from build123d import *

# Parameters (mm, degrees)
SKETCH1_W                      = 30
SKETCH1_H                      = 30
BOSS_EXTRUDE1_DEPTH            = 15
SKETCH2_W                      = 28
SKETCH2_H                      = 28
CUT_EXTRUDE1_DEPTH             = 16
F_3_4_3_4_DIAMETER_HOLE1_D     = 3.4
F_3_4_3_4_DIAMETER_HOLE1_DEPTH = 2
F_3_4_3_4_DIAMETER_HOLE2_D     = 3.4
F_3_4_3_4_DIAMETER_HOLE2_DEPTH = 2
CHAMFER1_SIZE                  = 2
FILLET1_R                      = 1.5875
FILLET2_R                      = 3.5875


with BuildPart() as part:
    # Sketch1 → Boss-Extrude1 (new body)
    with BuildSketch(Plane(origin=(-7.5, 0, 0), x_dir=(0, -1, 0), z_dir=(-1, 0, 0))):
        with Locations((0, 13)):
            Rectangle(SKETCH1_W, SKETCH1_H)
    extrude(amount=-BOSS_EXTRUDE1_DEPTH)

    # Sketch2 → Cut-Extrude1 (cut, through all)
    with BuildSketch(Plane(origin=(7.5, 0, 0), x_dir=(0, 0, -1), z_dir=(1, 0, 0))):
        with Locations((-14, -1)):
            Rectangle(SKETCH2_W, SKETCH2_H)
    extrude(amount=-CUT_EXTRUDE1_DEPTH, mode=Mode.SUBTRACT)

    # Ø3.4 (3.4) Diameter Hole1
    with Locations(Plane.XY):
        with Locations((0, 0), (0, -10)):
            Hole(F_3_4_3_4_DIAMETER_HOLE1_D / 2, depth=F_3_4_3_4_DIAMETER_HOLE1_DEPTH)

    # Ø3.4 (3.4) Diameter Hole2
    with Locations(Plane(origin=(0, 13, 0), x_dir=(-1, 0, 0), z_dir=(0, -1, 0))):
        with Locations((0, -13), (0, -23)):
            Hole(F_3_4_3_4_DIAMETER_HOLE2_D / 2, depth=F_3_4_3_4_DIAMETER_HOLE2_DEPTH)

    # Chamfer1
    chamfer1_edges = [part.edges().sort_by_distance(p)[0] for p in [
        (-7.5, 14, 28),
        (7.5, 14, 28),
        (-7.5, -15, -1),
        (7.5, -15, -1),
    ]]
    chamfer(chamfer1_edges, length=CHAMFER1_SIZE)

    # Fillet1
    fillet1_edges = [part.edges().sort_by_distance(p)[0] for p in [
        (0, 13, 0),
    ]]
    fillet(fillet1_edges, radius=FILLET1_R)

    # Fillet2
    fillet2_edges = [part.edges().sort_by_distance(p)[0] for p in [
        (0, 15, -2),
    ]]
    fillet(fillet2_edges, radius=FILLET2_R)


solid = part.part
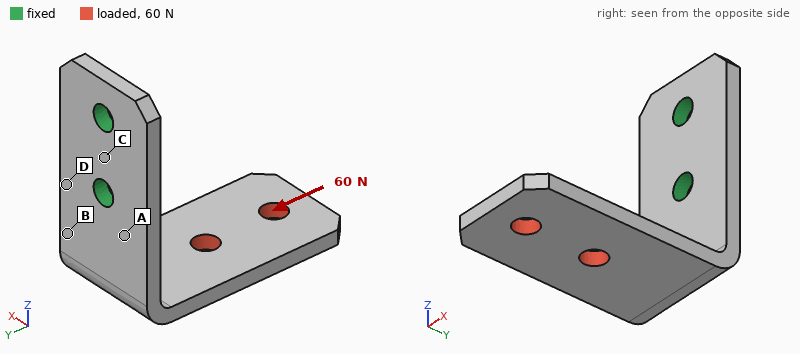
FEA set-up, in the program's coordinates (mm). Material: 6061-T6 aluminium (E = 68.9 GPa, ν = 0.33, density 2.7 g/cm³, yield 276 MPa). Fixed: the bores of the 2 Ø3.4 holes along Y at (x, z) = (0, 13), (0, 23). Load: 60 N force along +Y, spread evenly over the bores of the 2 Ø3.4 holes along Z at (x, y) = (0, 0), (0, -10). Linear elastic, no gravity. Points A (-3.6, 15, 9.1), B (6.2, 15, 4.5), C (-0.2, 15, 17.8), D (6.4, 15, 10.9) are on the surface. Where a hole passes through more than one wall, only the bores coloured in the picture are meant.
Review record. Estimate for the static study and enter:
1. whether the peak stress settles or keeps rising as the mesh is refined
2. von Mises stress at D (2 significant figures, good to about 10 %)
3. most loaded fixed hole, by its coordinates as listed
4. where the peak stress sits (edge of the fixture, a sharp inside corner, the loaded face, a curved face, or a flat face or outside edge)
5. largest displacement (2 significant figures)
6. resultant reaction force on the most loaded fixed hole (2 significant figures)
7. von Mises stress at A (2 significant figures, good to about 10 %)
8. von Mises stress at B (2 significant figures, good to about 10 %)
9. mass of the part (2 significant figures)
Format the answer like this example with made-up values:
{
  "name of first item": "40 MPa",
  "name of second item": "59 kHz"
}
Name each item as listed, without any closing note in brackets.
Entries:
{
  "whether the peak stress settles or keeps rising as the mesh is refined": "keeps rising",
  "von Mises stress at D": "45 MPa",
  "most loaded fixed hole, by its coordinates as listed": "(0, 13)",
  "where the peak stress sits": "edge of the fixture",
  "largest displacement": "0.23 mm",
  "resultant reaction force on the most loaded fixed hole": "77 N",
  "von Mises stress at A": "54 MPa",
  "von Mises stress at B": "33 MPa",
  "mass of the part": "4.4 g"
}
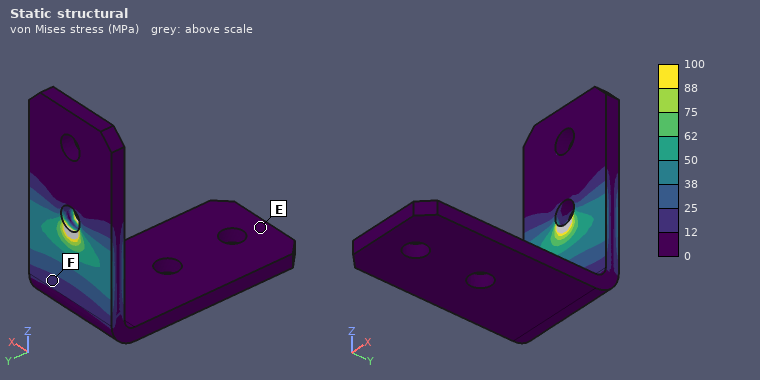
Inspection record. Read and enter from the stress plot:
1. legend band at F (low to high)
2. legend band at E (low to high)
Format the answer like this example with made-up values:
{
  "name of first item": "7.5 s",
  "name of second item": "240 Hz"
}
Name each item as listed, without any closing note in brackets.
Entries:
{
  "legend band at F": "12 to 25 MPa",
  "legend band at E": "0 to 12 MPa"
}
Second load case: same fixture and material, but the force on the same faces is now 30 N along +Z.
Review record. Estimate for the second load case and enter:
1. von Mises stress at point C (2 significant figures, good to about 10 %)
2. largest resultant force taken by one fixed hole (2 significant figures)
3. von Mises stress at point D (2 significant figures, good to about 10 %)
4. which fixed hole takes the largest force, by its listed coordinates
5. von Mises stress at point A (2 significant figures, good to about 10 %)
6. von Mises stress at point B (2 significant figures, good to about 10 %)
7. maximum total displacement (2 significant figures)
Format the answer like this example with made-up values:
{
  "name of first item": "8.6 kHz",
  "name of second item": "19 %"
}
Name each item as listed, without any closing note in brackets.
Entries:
{
  "von Mises stress at point C": "7.6 MPa",
  "largest resultant force taken by one fixed hole": "28 N",
  "von Mises stress at point D": "39 MPa",
  "which fixed hole takes the largest force, by its listed coordinates": "(0, 13)",
  "von Mises stress at point A": "51 MPa",
  "von Mises stress at point B": "57 MPa",
  "maximum total displacement": "0.47 mm"
}
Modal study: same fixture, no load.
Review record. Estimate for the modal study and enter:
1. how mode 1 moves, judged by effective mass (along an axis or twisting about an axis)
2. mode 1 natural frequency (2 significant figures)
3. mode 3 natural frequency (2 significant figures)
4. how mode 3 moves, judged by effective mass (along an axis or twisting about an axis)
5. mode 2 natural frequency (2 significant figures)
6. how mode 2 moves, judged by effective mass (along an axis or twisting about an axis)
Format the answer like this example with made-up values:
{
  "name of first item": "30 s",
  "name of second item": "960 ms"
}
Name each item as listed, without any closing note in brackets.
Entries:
{
  "how mode 1 moves, judged by effective mass": "along Z",
  "mode 1 natural frequency": "1200 Hz",
  "mode 3 natural frequency": "4300 Hz",
  "how mode 3 moves, judged by effective mass": "along Y",
  "mode 2 natural frequency": "1800 Hz",
  "how mode 2 moves, judged by effective mass": "along X"
}
